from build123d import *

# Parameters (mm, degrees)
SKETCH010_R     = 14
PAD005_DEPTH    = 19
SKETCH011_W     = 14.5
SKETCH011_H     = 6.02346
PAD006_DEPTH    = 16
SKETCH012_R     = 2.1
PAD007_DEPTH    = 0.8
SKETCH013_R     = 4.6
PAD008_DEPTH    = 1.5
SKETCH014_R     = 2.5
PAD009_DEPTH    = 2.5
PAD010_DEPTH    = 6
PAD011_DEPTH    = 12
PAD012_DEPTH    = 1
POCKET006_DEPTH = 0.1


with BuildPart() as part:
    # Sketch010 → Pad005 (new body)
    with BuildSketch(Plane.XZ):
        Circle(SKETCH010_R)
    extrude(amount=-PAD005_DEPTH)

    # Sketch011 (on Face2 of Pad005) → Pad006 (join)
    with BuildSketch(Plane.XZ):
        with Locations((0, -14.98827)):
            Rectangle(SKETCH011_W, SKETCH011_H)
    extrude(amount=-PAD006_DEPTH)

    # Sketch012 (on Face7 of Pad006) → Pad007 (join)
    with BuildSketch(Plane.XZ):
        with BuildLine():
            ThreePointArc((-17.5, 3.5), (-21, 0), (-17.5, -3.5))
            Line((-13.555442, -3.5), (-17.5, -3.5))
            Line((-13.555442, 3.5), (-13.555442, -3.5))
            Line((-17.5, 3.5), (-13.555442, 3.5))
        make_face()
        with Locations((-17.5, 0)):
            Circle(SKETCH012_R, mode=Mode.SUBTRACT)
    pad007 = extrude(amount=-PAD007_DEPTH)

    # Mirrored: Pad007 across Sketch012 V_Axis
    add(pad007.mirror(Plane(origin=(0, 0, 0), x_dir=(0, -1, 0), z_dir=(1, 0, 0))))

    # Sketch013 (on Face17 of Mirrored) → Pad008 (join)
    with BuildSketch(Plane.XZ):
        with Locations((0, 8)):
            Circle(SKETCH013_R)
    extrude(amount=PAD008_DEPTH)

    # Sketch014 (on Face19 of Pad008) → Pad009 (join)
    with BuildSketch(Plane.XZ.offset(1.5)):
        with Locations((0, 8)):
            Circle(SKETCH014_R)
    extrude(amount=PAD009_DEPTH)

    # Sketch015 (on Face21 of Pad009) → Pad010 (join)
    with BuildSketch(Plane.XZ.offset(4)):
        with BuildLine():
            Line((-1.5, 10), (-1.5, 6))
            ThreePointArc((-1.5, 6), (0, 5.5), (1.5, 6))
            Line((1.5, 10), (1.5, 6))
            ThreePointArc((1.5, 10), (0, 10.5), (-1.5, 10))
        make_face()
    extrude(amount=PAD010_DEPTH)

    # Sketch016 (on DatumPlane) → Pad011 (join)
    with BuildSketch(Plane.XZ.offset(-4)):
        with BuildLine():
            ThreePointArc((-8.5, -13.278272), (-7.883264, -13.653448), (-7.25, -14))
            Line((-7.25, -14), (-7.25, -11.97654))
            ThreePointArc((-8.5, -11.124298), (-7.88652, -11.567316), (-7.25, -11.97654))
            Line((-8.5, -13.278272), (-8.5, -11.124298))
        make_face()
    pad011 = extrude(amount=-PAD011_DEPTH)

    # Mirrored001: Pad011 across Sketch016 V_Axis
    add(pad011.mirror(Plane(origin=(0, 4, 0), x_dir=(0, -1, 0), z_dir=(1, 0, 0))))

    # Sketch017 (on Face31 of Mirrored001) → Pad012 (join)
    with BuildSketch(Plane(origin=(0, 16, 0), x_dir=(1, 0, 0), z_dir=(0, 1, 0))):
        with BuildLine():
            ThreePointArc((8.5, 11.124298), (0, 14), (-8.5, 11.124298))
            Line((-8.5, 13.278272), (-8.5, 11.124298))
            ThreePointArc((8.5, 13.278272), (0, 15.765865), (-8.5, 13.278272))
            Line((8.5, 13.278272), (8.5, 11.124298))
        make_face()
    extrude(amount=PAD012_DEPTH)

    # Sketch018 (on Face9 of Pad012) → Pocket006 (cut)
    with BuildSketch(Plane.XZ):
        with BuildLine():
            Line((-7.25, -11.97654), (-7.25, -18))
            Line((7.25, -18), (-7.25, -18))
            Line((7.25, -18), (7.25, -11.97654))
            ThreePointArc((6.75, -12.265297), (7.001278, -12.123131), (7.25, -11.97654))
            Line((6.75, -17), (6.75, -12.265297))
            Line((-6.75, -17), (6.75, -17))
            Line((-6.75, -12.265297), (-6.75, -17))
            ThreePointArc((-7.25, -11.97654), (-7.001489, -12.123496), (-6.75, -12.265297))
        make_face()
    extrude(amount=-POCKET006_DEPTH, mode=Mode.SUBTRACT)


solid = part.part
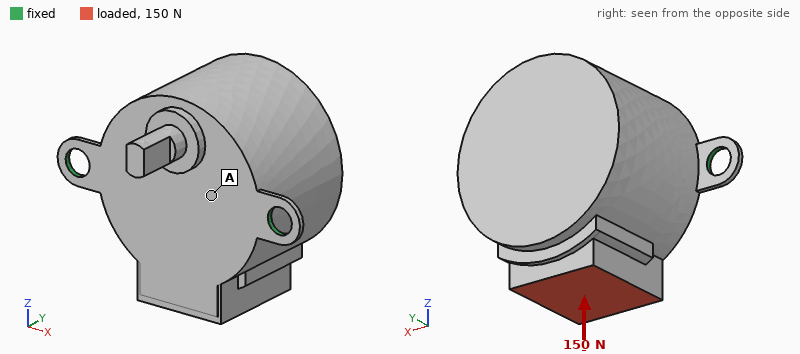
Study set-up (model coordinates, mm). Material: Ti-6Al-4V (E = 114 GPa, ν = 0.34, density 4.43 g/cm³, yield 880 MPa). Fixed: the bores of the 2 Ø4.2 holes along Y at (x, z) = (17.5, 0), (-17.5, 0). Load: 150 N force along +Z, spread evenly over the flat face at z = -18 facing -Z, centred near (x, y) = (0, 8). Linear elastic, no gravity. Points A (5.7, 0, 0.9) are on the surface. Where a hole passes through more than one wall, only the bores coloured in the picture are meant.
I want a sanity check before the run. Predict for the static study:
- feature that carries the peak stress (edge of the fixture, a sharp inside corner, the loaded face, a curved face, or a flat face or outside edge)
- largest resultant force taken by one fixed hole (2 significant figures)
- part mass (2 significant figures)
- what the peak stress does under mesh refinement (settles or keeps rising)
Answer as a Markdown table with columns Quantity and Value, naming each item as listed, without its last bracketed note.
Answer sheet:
| Quantity | Value |
|---|---|
| feature that carries the peak stress | edge of the fixture |
| largest resultant force taken by one fixed hole | 75 N |
| part mass | 58 g |
| what the peak stress does under mesh refinement | keeps rising |
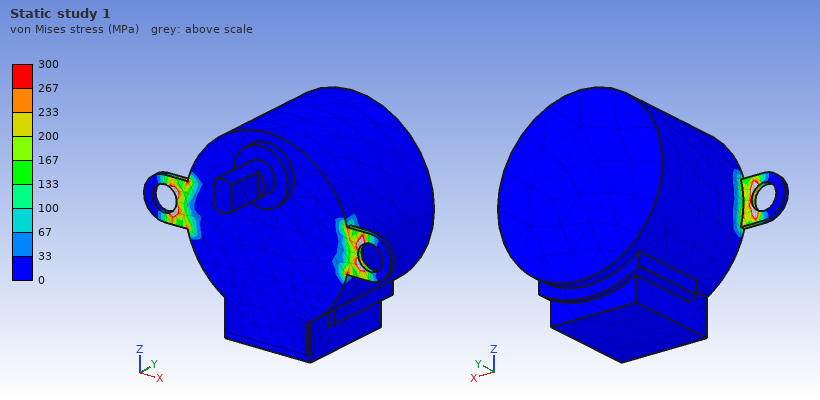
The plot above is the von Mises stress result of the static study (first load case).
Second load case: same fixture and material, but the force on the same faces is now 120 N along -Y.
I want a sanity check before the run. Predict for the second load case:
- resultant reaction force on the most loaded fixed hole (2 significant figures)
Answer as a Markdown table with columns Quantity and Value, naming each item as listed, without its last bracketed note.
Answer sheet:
| Quantity | Value |
|---|---|
| resultant reaction force on the most loaded fixed hole | 72 N |
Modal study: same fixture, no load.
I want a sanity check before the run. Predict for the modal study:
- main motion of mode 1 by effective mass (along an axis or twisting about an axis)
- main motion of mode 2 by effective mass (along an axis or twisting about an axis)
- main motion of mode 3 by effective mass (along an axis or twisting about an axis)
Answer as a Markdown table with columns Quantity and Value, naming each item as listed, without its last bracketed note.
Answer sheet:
| Quantity | Value |
|---|---|
| main motion of mode 1 by effective mass | along Z |
| main motion of mode 2 by effective mass | along Y |
| main motion of mode 3 by effective mass | along X |
